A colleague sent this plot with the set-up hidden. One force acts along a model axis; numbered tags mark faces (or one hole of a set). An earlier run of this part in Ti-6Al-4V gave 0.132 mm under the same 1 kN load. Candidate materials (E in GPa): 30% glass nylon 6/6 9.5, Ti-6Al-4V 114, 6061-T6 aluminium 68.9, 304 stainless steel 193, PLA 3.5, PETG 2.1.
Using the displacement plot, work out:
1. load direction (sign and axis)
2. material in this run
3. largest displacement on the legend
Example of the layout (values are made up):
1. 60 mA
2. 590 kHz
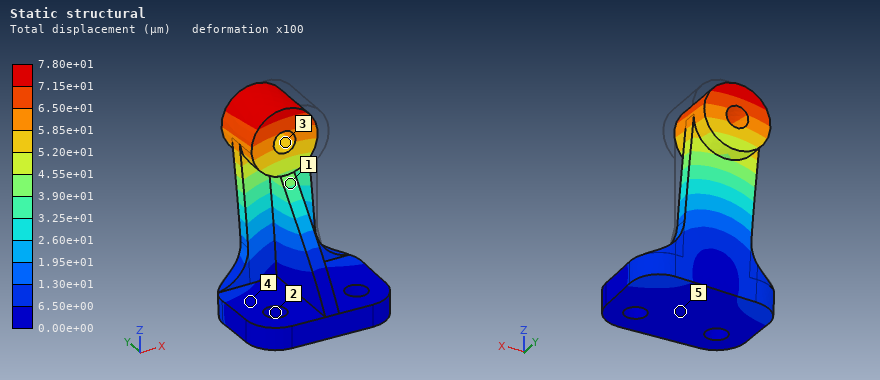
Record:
1. -X
2. 304 stainless steel
3. 7.80e+01 µm
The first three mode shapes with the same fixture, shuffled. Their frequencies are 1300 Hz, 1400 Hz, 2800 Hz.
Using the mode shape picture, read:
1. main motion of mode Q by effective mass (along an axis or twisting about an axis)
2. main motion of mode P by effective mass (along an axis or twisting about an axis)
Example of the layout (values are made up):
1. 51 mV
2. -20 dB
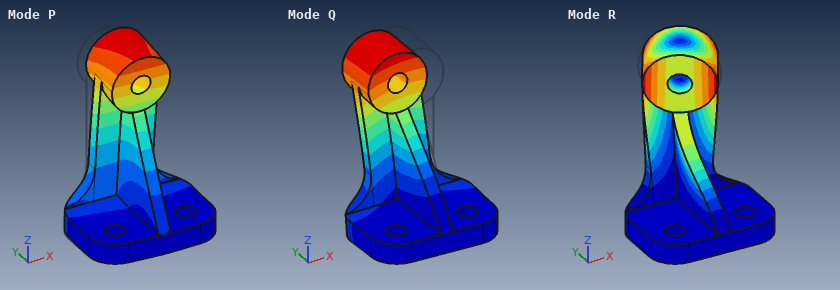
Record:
1. along X
2. along Y
